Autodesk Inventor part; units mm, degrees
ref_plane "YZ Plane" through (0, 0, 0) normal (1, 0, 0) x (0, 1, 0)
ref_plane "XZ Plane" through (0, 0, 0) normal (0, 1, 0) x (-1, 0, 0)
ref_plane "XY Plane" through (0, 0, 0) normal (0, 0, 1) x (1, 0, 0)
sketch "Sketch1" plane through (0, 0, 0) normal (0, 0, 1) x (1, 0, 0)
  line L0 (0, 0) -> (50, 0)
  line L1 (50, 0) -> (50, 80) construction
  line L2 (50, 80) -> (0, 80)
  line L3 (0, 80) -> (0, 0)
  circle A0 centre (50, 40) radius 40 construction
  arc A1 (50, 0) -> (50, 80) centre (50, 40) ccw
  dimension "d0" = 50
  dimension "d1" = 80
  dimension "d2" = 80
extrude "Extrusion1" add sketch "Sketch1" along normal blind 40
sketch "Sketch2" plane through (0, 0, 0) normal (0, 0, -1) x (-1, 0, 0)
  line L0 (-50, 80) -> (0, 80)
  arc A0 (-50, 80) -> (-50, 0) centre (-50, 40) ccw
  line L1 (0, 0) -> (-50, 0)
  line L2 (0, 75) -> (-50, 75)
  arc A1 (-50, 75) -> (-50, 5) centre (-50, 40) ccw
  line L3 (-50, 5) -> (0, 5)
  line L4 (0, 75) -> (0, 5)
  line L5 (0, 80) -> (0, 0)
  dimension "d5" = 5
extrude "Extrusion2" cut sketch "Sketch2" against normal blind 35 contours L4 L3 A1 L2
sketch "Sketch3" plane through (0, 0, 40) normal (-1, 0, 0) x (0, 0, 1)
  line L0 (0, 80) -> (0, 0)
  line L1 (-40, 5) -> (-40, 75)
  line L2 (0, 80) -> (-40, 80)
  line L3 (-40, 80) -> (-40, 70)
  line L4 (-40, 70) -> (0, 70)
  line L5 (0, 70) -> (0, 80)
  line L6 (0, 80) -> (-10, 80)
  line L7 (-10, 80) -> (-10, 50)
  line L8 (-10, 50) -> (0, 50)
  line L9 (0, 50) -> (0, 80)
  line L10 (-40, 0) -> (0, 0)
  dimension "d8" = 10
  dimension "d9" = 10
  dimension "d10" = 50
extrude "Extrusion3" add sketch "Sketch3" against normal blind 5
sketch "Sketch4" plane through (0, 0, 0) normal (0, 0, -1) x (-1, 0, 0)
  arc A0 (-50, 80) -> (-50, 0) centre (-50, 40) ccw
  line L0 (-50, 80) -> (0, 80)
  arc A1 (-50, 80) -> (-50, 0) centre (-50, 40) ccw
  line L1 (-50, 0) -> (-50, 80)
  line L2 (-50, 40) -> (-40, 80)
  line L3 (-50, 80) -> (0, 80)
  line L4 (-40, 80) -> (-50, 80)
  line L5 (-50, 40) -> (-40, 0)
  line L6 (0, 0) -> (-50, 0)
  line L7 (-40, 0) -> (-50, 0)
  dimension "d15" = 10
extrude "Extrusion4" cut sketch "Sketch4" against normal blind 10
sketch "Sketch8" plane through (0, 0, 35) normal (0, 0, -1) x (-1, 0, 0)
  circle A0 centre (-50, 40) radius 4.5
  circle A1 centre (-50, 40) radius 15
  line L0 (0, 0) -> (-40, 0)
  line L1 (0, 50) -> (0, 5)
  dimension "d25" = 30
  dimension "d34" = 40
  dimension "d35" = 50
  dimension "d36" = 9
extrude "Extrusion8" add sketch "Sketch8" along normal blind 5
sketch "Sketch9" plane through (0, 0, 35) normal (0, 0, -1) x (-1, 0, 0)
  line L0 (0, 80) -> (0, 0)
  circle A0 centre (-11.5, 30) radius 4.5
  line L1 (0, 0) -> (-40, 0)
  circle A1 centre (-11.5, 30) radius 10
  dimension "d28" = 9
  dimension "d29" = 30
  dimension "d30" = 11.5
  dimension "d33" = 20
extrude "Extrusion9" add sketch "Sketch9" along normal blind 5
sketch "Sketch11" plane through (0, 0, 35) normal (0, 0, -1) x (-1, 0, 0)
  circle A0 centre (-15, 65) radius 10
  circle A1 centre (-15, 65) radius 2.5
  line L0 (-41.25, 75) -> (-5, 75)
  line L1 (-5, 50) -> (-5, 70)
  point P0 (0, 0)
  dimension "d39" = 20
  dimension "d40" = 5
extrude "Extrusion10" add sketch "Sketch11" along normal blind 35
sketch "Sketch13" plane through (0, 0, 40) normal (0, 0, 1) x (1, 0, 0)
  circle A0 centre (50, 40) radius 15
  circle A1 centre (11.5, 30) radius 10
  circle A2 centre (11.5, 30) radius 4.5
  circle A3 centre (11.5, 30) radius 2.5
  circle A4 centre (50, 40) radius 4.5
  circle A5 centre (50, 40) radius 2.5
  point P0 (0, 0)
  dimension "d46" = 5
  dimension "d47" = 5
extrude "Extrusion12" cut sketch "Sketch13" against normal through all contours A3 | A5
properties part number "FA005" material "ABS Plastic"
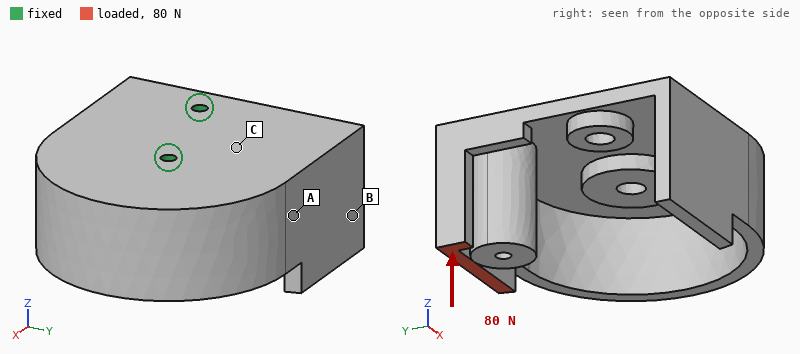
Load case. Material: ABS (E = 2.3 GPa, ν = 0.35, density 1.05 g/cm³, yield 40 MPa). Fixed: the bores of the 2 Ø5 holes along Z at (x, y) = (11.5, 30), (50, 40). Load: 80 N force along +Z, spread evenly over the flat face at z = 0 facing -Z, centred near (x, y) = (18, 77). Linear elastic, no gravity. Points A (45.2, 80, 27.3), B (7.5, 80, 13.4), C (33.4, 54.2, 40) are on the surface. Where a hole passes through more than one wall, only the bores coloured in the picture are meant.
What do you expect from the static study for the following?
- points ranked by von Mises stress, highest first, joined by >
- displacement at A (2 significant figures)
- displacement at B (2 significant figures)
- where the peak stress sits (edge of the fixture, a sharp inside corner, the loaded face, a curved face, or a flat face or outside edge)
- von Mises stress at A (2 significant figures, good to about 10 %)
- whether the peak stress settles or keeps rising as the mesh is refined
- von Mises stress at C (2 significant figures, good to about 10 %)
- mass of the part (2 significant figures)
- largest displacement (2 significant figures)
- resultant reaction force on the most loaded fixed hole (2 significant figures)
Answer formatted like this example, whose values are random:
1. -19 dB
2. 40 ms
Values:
1. C > A > B
2. 0.67 mm
3. 1.1 mm
4. edge of the fixture
5. 2.2 MPa
6. keeps rising
7. 4.2 MPa
8. 84 g
9. 1.4 mm
10. 42 N
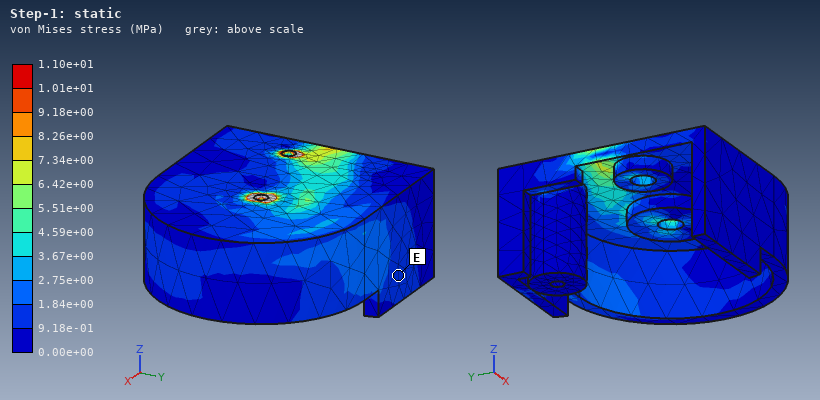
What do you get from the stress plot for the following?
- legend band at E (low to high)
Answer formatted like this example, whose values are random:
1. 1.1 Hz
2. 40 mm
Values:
1. 9.18e-01 to 1.84e+00 MPa
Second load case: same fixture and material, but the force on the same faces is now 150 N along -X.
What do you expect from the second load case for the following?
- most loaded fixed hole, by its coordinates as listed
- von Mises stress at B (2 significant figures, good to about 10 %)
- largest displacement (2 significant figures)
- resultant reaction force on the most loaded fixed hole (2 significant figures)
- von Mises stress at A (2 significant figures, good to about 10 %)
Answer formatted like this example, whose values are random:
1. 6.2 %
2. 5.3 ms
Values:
1. (50, 40)
2. 1.7 MPa
3. 1.3 mm
4. 220 N
5. 3.4 MPa
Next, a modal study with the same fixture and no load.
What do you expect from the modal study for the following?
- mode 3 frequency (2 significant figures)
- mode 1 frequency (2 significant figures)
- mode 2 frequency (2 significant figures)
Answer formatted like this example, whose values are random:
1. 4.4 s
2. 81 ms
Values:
1. 670 Hz
2. 270 Hz
3. 460 Hz
